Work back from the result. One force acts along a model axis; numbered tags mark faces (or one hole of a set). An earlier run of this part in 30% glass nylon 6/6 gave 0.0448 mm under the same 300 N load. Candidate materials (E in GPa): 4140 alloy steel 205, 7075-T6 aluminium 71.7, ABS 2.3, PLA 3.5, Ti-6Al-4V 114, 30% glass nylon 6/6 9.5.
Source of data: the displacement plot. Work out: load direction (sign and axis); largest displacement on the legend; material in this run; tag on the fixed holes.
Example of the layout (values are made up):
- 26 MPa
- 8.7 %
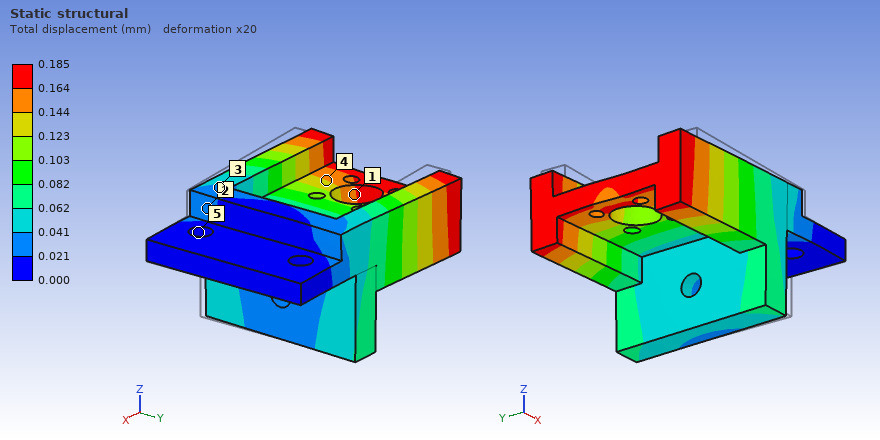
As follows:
- +Y
- 0.185 mm
- ABS
- 5
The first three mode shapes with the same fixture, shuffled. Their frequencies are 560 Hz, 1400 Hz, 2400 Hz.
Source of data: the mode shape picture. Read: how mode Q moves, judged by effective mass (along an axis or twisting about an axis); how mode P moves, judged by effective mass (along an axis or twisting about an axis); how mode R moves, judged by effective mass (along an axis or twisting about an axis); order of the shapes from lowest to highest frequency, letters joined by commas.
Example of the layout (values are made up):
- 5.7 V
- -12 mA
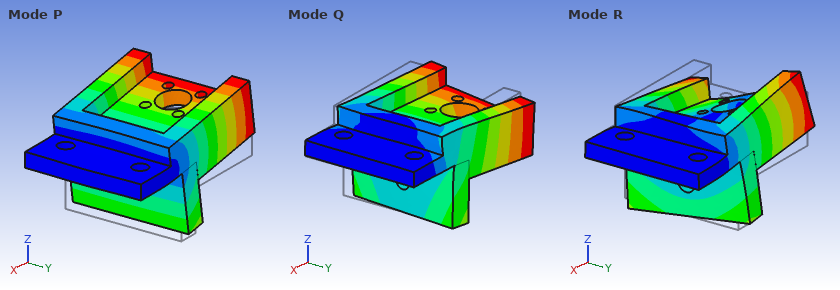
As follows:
- along Y
- along Z
- twisting about X
- P, R, Q
